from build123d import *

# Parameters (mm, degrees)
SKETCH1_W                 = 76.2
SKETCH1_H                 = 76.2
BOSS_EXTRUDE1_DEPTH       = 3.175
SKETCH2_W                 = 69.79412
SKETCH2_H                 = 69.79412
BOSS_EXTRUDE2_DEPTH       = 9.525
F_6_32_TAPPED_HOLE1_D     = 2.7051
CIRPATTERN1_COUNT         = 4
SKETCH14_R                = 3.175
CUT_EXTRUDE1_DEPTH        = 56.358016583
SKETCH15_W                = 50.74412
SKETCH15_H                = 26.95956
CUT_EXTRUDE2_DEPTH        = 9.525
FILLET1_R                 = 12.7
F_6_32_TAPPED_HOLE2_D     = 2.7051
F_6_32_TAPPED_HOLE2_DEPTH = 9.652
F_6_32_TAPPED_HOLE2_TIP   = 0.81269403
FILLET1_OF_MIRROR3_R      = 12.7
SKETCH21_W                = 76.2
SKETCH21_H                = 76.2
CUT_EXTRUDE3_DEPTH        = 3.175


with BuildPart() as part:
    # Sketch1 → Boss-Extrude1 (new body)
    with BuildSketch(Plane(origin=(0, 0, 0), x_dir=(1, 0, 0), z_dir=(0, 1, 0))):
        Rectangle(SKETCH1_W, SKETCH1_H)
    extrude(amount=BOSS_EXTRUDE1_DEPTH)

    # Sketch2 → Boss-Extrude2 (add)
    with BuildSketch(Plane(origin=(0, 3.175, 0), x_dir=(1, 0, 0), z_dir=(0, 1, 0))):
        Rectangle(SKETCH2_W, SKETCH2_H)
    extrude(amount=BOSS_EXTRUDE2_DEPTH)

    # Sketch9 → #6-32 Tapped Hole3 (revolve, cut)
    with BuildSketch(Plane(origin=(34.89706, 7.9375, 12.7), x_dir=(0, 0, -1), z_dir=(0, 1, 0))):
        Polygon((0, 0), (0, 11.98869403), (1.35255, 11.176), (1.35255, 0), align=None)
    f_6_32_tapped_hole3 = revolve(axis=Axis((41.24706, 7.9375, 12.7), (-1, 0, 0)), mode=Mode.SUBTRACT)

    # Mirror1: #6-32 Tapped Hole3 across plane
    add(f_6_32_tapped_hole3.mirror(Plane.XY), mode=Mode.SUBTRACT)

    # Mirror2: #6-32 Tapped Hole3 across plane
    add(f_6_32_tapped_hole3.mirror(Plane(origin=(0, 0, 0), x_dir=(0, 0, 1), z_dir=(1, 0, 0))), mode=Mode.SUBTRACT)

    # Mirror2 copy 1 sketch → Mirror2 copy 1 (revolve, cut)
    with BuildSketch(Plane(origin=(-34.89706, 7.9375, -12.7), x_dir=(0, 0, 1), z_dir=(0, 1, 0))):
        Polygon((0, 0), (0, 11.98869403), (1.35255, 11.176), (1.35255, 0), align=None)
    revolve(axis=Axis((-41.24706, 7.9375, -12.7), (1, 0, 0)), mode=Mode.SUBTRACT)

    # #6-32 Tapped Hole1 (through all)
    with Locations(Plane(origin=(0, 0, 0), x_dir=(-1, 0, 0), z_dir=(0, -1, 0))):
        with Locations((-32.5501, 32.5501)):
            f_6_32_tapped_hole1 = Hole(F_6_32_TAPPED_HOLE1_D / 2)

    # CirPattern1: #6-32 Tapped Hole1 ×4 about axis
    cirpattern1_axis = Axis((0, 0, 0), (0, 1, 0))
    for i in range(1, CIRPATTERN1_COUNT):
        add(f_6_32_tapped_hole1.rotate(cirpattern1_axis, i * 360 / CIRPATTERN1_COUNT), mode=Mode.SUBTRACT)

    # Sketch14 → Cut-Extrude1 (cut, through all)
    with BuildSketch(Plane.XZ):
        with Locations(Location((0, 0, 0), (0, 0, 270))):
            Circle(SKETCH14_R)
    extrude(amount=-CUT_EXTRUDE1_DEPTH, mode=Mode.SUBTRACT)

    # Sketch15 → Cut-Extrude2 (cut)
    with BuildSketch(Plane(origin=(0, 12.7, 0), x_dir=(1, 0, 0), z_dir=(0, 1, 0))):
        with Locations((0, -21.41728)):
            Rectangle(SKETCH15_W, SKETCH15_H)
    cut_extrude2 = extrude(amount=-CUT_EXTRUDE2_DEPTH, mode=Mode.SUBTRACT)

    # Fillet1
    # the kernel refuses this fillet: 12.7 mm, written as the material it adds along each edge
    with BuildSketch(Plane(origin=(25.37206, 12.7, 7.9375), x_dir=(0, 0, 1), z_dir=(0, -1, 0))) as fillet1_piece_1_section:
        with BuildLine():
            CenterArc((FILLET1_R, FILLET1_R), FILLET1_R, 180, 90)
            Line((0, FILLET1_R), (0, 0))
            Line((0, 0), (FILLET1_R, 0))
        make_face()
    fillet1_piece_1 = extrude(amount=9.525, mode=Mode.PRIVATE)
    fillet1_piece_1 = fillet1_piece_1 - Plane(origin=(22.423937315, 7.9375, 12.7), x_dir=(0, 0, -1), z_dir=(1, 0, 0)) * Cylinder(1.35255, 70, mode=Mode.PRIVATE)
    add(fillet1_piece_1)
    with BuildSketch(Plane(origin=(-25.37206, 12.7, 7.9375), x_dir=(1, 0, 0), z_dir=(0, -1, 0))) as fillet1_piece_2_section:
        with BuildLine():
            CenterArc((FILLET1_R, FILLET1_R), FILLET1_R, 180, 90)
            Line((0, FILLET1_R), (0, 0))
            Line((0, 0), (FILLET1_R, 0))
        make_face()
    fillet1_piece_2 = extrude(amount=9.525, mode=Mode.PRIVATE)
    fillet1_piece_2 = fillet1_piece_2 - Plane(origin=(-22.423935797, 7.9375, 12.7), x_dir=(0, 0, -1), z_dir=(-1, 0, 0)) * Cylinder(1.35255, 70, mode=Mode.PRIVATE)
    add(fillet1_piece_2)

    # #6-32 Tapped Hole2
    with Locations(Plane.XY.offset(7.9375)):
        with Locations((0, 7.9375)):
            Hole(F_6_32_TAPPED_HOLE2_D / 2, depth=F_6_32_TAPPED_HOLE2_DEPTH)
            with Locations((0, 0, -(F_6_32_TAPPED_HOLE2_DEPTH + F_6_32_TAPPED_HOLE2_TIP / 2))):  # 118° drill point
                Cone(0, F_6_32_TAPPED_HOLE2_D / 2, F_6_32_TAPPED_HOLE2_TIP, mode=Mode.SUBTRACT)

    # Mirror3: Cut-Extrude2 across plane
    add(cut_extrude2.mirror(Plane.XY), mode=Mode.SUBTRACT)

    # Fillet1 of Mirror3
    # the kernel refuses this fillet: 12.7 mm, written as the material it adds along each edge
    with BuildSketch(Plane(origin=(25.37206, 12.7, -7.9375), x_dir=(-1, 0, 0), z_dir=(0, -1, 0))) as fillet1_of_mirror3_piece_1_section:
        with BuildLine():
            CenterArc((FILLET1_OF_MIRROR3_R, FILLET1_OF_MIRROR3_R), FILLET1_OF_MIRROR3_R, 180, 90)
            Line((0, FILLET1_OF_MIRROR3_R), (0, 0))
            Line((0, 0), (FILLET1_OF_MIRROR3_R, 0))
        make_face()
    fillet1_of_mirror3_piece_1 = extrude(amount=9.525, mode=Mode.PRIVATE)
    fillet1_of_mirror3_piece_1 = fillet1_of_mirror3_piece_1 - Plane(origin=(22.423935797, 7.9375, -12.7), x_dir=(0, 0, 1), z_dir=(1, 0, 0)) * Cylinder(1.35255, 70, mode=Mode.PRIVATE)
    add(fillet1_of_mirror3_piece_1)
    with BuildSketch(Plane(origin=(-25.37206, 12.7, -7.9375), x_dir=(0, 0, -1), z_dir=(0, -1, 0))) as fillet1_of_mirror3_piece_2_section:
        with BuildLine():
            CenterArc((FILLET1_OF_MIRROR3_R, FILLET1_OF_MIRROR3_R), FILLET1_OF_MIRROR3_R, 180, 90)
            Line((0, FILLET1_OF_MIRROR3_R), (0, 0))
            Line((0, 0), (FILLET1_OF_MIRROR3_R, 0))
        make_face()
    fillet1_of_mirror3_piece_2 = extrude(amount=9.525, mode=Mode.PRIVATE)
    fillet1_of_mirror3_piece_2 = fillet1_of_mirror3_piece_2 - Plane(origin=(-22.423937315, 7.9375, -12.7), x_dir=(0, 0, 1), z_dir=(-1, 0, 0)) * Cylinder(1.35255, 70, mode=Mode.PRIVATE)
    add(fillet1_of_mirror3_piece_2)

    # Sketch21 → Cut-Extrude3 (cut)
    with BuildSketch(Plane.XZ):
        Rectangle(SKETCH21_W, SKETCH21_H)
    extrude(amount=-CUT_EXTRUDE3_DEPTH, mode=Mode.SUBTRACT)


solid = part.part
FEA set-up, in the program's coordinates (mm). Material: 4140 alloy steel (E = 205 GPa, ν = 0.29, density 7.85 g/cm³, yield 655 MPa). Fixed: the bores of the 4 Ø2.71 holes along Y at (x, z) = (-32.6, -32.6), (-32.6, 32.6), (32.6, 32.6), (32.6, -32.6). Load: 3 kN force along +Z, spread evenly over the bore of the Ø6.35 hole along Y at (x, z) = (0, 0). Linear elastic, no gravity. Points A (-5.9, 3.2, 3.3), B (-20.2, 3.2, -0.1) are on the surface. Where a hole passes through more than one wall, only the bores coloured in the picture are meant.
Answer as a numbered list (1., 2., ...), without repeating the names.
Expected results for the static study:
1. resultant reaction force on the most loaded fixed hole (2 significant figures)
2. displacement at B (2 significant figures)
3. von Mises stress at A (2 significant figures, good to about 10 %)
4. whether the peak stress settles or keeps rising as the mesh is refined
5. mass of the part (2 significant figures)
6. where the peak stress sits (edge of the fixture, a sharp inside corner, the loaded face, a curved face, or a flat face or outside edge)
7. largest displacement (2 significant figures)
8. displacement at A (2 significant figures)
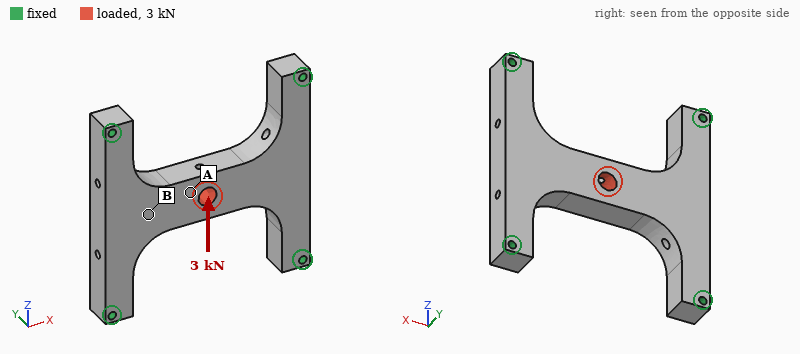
1. 890 N
2. 3.0 µm
3. 27 MPa
4. keeps rising
5. 160 g
6. a sharp inside corner
7. 9.6 µm
8. 8.3 µm
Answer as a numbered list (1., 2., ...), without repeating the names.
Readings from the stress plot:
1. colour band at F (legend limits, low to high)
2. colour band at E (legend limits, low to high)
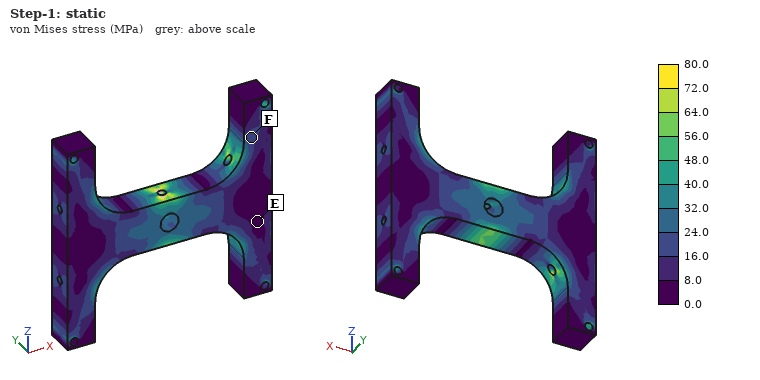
1. 16.0 to 24.0 MPa
2. 0.0 to 8.0 MPa
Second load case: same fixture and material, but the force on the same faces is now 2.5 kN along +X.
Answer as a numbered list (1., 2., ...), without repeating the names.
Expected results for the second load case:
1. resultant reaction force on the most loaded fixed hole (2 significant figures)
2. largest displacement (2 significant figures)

1. 1.0 kN
2. 9.8 µm
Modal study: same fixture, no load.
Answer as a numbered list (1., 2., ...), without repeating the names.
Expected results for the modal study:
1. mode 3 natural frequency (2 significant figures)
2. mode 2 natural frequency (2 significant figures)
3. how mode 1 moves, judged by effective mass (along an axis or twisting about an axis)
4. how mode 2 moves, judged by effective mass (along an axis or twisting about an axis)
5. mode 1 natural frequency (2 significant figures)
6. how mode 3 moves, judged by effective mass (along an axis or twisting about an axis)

1. 9100 Hz
2. 7700 Hz
3. along Y
4. along X
5. 5400 Hz
6. twisting about Z
